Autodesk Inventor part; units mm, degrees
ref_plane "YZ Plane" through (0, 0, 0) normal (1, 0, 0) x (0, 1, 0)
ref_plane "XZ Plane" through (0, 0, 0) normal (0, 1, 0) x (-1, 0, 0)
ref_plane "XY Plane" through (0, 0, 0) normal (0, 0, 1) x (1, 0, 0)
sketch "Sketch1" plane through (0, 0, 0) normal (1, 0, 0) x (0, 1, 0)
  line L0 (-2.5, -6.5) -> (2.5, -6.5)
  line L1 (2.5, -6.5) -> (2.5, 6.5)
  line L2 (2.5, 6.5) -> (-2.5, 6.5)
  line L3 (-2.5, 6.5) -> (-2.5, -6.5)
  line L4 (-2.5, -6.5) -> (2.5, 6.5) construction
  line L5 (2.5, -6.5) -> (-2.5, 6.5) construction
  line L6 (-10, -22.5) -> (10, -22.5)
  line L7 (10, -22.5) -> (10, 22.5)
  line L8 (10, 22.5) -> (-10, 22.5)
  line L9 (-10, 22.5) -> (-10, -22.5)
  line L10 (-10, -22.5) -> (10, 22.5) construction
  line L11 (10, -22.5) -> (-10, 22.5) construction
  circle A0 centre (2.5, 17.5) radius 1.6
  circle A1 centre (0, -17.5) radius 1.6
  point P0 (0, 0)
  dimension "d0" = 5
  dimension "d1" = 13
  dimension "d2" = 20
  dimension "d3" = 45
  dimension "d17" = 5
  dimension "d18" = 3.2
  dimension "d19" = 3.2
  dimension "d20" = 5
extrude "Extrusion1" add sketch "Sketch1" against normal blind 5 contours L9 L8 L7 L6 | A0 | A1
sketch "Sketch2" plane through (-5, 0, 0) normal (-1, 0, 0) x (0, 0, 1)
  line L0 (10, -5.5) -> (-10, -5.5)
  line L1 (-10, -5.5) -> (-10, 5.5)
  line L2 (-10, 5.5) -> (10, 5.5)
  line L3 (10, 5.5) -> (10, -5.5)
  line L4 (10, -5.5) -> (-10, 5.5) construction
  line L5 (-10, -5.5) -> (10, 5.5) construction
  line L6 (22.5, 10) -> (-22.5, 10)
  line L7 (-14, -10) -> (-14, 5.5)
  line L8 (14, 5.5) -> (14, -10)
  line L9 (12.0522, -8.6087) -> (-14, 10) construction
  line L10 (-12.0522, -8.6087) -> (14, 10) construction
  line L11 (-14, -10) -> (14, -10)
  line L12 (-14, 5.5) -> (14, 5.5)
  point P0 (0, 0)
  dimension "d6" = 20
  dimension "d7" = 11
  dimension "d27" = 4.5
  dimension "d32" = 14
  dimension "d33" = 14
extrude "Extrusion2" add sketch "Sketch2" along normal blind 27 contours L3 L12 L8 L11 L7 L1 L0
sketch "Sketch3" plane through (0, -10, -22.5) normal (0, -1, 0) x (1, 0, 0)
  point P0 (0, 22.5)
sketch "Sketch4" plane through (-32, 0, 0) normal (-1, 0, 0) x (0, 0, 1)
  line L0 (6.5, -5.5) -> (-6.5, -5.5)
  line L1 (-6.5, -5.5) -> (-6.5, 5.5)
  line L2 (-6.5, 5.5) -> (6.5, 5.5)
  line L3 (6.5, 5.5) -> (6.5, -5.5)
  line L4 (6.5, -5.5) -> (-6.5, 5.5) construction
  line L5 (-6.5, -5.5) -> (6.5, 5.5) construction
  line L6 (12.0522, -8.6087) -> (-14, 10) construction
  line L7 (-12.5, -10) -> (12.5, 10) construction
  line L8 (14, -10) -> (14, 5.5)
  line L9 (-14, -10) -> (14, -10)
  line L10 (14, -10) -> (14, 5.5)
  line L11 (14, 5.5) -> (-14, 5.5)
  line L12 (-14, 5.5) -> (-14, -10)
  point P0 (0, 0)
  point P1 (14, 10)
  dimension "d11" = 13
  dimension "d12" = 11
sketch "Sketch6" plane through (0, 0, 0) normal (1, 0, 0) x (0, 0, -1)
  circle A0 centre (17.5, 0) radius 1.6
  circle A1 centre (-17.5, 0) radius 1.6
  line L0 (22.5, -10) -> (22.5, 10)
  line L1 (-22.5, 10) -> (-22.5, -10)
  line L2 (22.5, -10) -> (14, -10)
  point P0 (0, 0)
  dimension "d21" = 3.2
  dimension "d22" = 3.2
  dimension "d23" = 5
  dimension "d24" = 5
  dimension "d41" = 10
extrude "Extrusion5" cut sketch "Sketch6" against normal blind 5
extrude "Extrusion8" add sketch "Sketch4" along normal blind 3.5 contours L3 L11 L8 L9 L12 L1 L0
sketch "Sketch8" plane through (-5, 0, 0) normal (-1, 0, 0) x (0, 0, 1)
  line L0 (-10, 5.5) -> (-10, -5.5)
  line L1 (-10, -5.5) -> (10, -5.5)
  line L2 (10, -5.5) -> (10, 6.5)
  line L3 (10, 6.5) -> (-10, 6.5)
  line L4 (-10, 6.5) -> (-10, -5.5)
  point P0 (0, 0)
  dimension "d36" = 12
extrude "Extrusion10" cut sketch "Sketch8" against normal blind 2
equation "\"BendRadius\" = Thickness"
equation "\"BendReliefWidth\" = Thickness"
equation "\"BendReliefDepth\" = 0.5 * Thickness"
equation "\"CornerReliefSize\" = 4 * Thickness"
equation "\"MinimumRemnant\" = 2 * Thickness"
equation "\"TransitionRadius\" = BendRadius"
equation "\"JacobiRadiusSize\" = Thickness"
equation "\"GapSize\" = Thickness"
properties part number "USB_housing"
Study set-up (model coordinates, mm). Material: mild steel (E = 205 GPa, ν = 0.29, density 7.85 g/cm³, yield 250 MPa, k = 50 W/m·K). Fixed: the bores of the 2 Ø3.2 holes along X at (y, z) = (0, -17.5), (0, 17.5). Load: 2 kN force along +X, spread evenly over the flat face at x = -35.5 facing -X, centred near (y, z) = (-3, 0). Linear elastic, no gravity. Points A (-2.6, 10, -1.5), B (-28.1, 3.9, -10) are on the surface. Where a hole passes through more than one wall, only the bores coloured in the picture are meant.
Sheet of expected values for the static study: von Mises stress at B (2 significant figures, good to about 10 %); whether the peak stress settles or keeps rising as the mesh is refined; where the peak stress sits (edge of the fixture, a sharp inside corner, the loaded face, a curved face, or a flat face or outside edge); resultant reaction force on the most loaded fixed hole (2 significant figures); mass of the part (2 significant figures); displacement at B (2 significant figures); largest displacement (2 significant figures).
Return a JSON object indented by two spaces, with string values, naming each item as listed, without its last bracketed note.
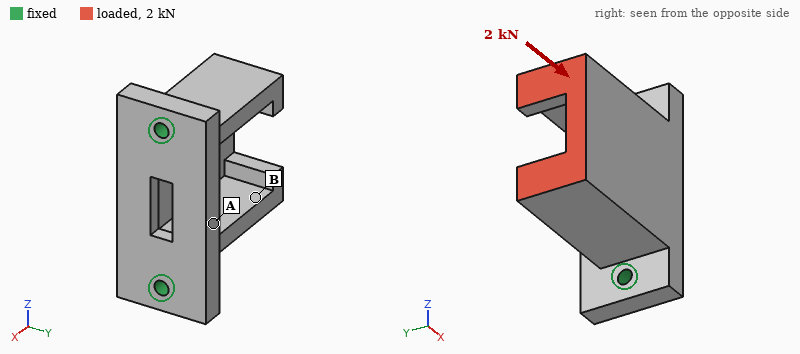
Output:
{
  "von Mises stress at B": "25 MPa",
  "whether the peak stress settles or keeps rising as the mesh is refined": "keeps rising",
  "where the peak stress sits": "edge of the fixture",
  "resultant reaction force on the most loaded fixed hole": "1.0 kN",
  "mass of the part": "83 g",
  "displacement at B": "9.8 µm",
  "largest displacement": "15 µm"
}
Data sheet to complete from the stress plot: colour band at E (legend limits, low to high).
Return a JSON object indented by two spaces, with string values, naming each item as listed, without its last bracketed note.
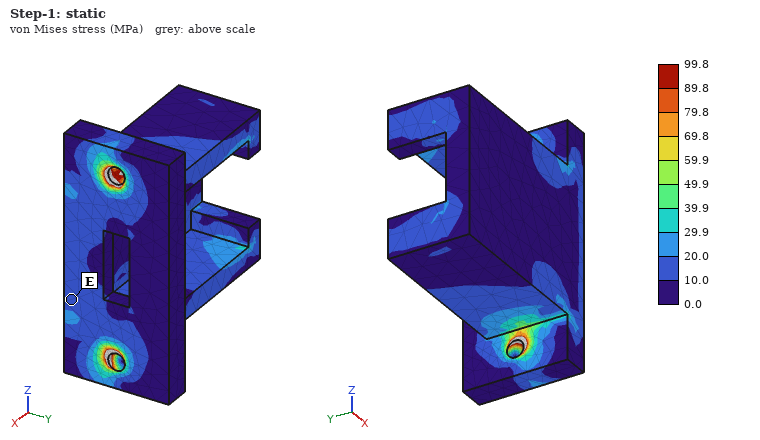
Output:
{
  "colour band at E": "10.0 to 20.0 MPa"
}
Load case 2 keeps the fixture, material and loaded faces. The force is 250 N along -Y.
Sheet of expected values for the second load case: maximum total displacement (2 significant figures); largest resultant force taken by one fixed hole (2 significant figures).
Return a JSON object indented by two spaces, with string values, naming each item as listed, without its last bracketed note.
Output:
{
  "maximum total displacement": "22 µm",
  "largest resultant force taken by one fixed hole": "130 N"
}
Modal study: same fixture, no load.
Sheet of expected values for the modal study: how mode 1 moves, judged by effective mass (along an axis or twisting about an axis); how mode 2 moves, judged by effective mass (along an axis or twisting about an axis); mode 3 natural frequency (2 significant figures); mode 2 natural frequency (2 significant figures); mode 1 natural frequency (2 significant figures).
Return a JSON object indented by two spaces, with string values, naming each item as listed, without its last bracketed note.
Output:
{
  "how mode 1 moves, judged by effective mass": "along Y",
  "how mode 2 moves, judged by effective mass": "along Z",
  "mode 3 natural frequency": "13 kHz",
  "mode 2 natural frequency": "5900 Hz",
  "mode 1 natural frequency": "3800 Hz"
}
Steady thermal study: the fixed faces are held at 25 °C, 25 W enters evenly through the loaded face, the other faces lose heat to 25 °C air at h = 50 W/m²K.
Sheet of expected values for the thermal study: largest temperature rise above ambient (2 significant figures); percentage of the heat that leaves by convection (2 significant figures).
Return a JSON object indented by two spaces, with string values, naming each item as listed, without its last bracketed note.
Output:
{
  "largest temperature rise above ambient": "79 K",
  "percentage of the heat that leaves by convection": "35 %"
}
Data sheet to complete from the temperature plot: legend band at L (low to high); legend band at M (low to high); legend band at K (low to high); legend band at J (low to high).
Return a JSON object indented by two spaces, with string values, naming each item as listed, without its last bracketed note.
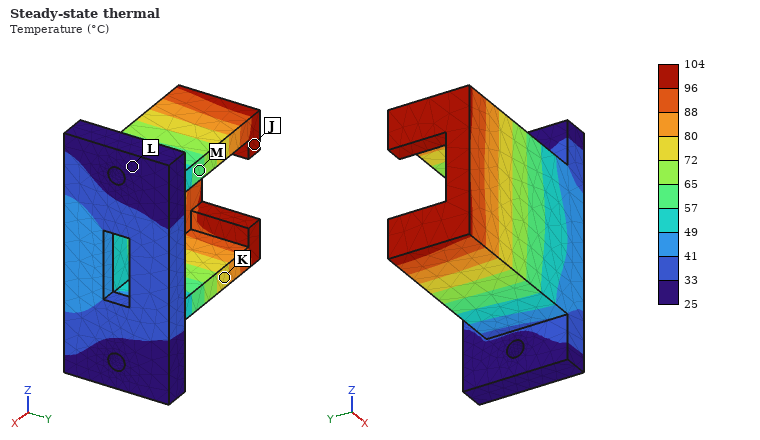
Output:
{
  "legend band at L": "25 to 33 °C",
  "legend band at M": "57 to 65 °C",
  "legend band at K": "72 to 80 °C",
  "legend band at J": "96 to 104 °C"
}
